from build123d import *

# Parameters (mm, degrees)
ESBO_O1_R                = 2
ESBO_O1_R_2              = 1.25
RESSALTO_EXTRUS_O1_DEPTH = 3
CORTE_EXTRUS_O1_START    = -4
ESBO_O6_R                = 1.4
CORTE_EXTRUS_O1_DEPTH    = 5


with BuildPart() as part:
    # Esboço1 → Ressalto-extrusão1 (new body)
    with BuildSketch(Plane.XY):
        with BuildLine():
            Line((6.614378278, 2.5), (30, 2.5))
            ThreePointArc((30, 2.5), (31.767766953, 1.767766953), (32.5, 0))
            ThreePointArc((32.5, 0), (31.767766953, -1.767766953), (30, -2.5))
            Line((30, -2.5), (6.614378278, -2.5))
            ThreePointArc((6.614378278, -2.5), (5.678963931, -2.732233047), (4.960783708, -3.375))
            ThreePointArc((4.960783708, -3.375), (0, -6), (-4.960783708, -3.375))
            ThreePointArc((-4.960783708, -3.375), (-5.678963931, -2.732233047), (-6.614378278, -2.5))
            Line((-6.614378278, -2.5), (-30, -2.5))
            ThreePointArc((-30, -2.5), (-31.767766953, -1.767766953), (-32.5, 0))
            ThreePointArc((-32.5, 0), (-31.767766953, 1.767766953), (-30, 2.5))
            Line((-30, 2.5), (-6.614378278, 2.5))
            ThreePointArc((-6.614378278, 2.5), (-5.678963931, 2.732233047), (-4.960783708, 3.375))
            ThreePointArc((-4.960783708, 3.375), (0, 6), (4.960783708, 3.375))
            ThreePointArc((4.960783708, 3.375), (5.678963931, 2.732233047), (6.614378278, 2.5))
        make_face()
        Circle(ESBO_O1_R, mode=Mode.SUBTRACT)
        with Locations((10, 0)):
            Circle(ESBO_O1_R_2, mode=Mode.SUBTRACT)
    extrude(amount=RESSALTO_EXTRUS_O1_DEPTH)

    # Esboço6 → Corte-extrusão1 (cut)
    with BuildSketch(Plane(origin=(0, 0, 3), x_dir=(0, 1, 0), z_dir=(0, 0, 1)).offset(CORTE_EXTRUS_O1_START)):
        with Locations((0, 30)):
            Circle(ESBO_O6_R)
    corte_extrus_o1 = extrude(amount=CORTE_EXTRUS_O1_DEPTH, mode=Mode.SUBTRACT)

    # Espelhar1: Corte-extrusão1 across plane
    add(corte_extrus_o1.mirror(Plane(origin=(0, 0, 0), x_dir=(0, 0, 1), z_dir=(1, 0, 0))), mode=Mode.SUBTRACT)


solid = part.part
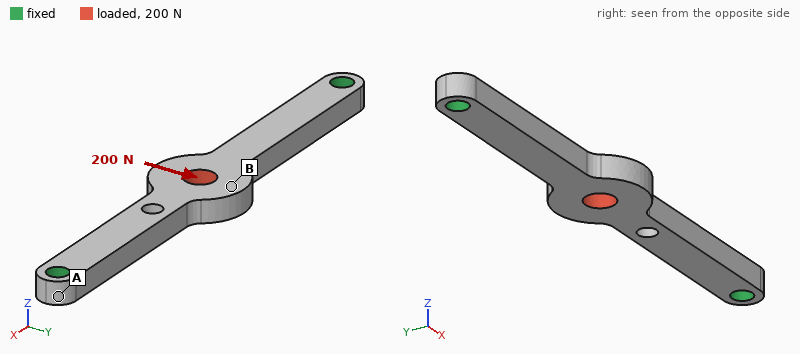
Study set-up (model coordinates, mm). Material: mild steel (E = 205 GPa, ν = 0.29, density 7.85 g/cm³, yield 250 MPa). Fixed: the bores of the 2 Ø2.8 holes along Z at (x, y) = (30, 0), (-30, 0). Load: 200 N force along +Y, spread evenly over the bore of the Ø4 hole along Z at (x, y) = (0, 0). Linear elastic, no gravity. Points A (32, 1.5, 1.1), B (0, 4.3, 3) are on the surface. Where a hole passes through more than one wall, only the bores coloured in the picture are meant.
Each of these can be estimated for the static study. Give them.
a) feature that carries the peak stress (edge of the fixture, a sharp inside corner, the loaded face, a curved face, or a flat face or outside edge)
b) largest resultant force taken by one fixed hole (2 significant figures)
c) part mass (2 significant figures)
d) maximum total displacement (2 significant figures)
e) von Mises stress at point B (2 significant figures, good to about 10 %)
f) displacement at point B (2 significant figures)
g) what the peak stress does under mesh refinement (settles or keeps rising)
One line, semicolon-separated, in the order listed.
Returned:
edge of the fixture; 100 N; 8.1 g; 26 µm; 18 MPa; 26 µm; keeps rising
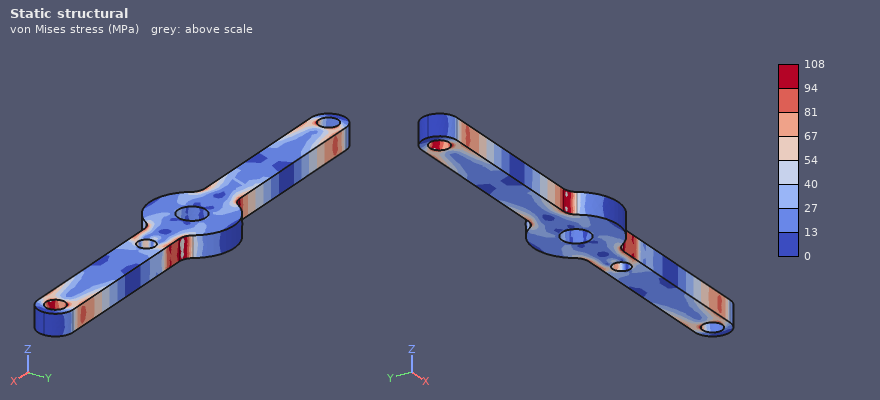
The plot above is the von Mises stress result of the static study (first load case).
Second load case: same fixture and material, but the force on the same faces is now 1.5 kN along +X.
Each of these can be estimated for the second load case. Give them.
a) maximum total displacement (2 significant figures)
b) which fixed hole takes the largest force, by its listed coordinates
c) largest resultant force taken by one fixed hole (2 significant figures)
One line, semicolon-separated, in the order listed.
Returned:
7.3 µm; (-30, 0); 800 N
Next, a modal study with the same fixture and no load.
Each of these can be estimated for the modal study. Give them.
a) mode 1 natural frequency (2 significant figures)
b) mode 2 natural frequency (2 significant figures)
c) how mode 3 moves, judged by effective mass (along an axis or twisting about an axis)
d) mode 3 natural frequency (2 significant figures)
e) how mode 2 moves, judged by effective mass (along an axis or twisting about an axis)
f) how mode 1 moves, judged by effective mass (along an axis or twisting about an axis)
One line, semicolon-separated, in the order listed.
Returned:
4000 Hz; 6800 Hz; twisting about Y; 12 kHz; along Y; along Z
